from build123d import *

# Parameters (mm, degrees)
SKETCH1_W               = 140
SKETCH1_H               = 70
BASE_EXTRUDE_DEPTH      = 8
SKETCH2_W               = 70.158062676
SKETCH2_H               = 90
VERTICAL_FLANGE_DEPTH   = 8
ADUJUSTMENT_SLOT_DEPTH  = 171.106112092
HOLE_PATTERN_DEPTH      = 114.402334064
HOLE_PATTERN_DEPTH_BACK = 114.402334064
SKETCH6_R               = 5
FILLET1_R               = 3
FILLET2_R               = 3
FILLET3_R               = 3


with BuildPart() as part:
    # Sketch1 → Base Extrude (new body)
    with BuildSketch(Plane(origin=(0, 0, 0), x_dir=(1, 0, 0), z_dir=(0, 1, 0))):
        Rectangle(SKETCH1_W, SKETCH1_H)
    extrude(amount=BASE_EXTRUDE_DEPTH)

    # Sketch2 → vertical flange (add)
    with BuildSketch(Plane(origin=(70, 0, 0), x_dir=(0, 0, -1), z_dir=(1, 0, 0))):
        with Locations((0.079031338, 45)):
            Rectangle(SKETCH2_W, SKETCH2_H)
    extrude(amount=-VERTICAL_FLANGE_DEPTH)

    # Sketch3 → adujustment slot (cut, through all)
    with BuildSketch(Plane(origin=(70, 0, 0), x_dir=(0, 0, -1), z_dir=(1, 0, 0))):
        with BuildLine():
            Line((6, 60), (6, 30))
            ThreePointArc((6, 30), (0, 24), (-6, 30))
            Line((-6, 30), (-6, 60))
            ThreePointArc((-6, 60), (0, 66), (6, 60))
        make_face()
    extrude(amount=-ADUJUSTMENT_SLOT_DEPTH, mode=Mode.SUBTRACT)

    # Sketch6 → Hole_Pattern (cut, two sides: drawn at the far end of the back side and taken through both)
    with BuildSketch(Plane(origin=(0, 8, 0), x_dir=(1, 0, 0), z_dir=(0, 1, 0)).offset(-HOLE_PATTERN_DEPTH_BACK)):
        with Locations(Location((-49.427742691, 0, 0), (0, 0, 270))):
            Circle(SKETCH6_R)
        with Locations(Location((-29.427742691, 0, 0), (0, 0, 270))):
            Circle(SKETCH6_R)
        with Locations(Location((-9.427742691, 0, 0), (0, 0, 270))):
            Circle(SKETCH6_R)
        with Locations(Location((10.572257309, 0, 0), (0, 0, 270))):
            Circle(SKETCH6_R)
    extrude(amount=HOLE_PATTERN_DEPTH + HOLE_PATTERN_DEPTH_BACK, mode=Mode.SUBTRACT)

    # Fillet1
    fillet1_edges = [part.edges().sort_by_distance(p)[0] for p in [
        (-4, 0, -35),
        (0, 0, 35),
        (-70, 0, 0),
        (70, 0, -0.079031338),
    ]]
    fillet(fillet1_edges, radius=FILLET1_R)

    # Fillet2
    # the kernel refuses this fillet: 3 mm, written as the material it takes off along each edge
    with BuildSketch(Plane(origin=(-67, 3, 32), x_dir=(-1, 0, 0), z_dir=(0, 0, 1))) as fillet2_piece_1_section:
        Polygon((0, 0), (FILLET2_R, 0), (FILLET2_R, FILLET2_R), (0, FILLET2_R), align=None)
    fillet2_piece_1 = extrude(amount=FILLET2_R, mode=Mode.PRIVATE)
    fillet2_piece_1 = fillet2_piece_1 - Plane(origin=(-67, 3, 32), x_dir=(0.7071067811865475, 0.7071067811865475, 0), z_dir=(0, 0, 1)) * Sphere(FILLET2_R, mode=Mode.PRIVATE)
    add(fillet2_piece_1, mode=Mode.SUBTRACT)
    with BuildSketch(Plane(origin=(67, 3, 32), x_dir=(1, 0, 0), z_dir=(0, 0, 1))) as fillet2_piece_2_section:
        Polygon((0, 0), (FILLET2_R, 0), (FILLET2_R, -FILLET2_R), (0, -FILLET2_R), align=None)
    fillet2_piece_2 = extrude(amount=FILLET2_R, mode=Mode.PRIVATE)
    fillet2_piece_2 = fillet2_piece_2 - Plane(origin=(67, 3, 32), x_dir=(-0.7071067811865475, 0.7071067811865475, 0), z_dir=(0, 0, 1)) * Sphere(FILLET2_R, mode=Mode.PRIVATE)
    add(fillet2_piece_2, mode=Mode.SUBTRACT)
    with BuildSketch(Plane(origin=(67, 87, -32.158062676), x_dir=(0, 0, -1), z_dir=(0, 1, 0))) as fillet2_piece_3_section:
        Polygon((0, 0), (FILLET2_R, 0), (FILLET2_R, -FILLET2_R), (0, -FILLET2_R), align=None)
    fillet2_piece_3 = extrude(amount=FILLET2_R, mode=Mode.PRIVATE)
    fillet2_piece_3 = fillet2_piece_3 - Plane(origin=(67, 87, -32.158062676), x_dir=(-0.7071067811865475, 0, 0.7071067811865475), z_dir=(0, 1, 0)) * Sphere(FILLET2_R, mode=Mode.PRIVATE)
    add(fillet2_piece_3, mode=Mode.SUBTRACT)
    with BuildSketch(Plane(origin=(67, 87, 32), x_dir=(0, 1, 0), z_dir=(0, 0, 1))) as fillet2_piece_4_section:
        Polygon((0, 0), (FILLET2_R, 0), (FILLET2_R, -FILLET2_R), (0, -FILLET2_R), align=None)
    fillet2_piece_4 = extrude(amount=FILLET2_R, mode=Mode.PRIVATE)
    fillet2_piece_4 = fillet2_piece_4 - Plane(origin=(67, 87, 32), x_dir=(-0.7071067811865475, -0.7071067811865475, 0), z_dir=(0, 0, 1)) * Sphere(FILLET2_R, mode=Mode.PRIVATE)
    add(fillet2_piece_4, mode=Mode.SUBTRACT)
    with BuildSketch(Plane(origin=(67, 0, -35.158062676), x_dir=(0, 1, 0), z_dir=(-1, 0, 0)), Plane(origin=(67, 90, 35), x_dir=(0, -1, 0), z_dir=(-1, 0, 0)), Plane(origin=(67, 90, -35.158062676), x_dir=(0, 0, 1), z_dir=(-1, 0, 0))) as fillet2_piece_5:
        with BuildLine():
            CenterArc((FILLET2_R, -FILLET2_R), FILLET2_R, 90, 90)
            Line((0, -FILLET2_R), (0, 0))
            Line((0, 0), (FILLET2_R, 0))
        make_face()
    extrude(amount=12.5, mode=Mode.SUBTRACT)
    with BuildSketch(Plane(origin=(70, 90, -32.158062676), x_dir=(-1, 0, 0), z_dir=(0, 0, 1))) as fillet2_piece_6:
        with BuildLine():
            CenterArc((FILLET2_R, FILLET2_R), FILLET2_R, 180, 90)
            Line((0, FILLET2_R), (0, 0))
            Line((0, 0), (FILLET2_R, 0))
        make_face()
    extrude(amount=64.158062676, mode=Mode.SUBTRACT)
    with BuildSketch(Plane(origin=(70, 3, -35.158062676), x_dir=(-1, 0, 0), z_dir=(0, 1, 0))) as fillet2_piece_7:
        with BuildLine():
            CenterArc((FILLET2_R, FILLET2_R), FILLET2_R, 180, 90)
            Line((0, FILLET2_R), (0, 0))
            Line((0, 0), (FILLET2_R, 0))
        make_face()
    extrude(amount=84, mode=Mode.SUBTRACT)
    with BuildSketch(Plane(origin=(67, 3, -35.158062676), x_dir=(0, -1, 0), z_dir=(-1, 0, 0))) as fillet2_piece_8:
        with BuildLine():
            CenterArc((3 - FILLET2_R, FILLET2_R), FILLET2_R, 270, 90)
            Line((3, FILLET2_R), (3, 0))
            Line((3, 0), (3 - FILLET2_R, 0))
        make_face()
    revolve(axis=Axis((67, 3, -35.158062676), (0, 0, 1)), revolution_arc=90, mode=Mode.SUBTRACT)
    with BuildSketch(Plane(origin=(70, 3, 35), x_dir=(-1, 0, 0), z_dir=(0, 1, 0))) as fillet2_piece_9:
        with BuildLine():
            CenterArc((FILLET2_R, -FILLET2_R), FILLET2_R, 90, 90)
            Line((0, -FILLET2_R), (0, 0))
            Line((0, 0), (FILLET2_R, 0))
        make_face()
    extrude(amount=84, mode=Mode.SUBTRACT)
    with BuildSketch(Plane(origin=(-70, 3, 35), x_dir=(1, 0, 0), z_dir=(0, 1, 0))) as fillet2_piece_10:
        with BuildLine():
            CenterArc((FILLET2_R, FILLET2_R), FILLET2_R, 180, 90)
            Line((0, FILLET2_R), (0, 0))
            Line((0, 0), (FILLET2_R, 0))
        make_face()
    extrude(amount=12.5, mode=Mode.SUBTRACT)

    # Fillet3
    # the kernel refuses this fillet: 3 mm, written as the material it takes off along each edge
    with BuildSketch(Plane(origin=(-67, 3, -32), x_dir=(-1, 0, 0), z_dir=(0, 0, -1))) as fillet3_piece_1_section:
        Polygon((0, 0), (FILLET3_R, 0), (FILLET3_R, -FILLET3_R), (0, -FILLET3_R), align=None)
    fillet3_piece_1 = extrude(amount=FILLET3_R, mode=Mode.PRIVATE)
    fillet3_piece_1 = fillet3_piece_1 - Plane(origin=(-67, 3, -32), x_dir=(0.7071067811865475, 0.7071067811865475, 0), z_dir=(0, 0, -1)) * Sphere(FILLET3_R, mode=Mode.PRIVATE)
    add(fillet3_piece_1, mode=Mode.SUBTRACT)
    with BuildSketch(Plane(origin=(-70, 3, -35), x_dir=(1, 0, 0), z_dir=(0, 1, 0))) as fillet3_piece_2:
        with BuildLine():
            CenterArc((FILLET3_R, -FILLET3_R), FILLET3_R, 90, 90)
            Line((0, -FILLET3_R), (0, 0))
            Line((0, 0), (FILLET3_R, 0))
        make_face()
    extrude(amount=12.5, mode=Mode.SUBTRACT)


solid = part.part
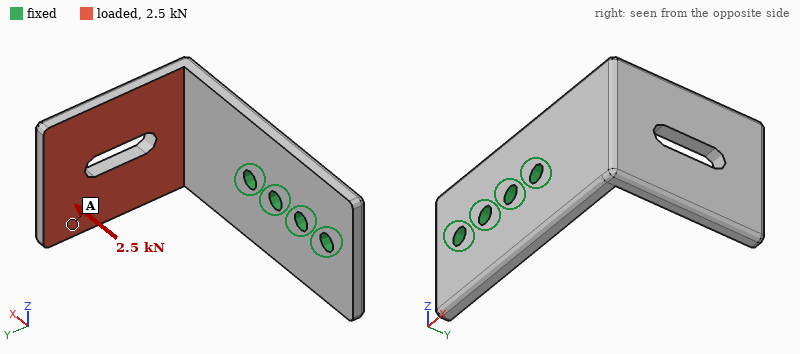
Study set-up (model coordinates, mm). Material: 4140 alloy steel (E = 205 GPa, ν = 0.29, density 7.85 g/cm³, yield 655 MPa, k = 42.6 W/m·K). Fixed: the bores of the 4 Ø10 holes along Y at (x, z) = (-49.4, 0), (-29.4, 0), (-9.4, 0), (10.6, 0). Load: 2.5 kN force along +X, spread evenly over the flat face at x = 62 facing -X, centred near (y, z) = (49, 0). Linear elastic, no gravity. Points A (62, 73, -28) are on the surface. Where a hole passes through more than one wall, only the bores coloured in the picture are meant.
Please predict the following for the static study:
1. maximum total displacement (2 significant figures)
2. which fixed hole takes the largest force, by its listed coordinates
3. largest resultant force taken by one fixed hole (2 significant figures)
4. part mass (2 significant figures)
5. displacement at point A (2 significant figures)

1.2 mm
(10.6, 0)
2.6 kN
920 g
0.96 mm
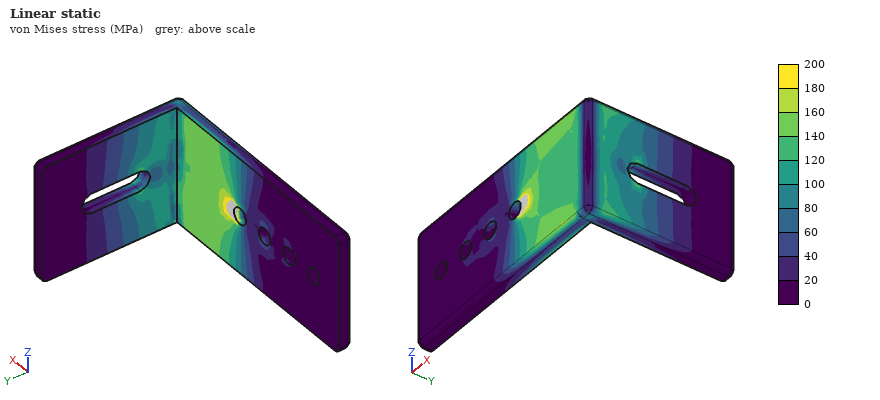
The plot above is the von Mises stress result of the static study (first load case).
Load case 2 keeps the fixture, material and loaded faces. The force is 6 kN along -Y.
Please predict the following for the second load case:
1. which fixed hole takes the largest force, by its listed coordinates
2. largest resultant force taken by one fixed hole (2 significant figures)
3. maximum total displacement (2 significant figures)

(10.6, 0)
11 kN
1.2 mm
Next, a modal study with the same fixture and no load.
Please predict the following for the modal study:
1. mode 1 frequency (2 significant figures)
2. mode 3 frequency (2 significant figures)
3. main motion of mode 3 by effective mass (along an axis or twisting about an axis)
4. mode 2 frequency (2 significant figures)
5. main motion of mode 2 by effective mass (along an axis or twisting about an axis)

440 Hz
1300 Hz
along Y
660 Hz
along Z
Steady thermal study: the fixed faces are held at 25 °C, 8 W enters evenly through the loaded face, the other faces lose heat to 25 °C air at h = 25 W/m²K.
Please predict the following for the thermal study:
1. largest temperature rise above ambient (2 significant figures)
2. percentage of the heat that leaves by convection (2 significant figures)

19 K
56 %
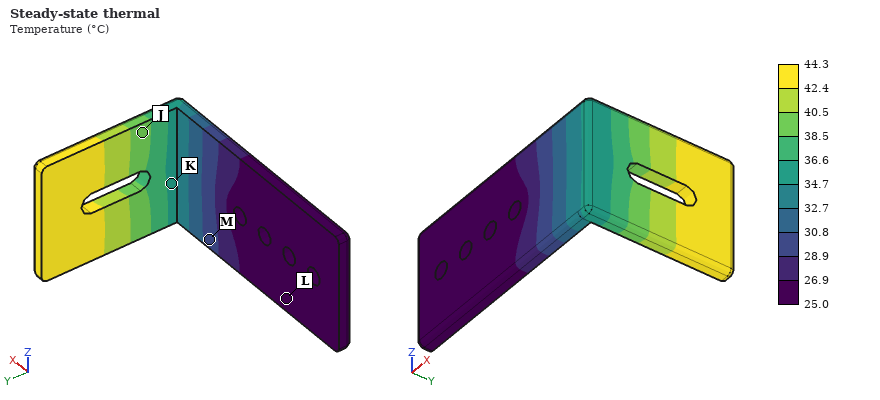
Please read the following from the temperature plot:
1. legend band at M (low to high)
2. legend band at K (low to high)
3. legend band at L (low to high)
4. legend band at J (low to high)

28.9 to 30.8 °C
34.7 to 36.6 °C
25.0 to 26.9 °C
38.5 to 40.5 °C
